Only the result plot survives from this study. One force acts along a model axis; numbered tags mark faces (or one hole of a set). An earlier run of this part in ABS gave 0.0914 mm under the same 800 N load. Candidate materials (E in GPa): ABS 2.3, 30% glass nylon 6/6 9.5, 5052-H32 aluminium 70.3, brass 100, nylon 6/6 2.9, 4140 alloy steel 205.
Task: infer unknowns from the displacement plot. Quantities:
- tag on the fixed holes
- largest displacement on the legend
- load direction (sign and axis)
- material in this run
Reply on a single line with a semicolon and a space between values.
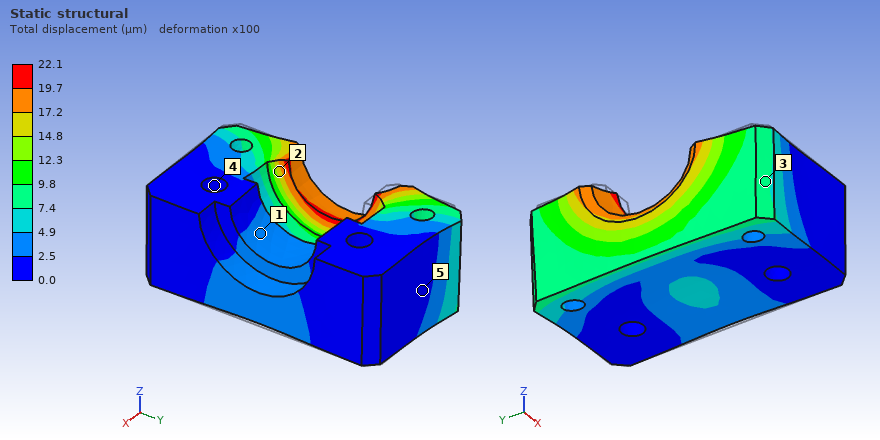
4; 22.1 µm; -X; 30% glass nylon 6/6
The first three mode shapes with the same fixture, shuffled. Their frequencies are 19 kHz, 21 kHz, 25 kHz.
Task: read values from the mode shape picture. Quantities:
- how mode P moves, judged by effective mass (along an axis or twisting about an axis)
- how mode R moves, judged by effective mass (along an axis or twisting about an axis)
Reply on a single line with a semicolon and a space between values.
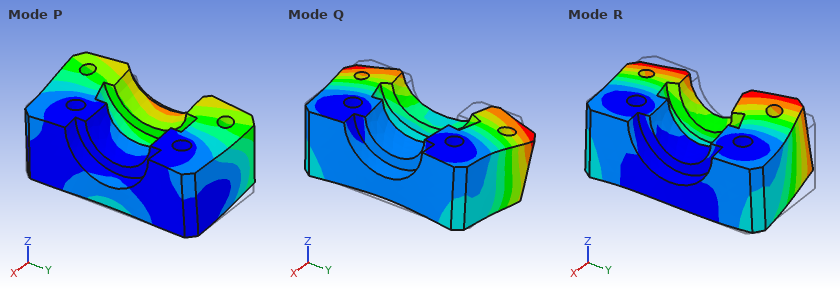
along Z; along Y
